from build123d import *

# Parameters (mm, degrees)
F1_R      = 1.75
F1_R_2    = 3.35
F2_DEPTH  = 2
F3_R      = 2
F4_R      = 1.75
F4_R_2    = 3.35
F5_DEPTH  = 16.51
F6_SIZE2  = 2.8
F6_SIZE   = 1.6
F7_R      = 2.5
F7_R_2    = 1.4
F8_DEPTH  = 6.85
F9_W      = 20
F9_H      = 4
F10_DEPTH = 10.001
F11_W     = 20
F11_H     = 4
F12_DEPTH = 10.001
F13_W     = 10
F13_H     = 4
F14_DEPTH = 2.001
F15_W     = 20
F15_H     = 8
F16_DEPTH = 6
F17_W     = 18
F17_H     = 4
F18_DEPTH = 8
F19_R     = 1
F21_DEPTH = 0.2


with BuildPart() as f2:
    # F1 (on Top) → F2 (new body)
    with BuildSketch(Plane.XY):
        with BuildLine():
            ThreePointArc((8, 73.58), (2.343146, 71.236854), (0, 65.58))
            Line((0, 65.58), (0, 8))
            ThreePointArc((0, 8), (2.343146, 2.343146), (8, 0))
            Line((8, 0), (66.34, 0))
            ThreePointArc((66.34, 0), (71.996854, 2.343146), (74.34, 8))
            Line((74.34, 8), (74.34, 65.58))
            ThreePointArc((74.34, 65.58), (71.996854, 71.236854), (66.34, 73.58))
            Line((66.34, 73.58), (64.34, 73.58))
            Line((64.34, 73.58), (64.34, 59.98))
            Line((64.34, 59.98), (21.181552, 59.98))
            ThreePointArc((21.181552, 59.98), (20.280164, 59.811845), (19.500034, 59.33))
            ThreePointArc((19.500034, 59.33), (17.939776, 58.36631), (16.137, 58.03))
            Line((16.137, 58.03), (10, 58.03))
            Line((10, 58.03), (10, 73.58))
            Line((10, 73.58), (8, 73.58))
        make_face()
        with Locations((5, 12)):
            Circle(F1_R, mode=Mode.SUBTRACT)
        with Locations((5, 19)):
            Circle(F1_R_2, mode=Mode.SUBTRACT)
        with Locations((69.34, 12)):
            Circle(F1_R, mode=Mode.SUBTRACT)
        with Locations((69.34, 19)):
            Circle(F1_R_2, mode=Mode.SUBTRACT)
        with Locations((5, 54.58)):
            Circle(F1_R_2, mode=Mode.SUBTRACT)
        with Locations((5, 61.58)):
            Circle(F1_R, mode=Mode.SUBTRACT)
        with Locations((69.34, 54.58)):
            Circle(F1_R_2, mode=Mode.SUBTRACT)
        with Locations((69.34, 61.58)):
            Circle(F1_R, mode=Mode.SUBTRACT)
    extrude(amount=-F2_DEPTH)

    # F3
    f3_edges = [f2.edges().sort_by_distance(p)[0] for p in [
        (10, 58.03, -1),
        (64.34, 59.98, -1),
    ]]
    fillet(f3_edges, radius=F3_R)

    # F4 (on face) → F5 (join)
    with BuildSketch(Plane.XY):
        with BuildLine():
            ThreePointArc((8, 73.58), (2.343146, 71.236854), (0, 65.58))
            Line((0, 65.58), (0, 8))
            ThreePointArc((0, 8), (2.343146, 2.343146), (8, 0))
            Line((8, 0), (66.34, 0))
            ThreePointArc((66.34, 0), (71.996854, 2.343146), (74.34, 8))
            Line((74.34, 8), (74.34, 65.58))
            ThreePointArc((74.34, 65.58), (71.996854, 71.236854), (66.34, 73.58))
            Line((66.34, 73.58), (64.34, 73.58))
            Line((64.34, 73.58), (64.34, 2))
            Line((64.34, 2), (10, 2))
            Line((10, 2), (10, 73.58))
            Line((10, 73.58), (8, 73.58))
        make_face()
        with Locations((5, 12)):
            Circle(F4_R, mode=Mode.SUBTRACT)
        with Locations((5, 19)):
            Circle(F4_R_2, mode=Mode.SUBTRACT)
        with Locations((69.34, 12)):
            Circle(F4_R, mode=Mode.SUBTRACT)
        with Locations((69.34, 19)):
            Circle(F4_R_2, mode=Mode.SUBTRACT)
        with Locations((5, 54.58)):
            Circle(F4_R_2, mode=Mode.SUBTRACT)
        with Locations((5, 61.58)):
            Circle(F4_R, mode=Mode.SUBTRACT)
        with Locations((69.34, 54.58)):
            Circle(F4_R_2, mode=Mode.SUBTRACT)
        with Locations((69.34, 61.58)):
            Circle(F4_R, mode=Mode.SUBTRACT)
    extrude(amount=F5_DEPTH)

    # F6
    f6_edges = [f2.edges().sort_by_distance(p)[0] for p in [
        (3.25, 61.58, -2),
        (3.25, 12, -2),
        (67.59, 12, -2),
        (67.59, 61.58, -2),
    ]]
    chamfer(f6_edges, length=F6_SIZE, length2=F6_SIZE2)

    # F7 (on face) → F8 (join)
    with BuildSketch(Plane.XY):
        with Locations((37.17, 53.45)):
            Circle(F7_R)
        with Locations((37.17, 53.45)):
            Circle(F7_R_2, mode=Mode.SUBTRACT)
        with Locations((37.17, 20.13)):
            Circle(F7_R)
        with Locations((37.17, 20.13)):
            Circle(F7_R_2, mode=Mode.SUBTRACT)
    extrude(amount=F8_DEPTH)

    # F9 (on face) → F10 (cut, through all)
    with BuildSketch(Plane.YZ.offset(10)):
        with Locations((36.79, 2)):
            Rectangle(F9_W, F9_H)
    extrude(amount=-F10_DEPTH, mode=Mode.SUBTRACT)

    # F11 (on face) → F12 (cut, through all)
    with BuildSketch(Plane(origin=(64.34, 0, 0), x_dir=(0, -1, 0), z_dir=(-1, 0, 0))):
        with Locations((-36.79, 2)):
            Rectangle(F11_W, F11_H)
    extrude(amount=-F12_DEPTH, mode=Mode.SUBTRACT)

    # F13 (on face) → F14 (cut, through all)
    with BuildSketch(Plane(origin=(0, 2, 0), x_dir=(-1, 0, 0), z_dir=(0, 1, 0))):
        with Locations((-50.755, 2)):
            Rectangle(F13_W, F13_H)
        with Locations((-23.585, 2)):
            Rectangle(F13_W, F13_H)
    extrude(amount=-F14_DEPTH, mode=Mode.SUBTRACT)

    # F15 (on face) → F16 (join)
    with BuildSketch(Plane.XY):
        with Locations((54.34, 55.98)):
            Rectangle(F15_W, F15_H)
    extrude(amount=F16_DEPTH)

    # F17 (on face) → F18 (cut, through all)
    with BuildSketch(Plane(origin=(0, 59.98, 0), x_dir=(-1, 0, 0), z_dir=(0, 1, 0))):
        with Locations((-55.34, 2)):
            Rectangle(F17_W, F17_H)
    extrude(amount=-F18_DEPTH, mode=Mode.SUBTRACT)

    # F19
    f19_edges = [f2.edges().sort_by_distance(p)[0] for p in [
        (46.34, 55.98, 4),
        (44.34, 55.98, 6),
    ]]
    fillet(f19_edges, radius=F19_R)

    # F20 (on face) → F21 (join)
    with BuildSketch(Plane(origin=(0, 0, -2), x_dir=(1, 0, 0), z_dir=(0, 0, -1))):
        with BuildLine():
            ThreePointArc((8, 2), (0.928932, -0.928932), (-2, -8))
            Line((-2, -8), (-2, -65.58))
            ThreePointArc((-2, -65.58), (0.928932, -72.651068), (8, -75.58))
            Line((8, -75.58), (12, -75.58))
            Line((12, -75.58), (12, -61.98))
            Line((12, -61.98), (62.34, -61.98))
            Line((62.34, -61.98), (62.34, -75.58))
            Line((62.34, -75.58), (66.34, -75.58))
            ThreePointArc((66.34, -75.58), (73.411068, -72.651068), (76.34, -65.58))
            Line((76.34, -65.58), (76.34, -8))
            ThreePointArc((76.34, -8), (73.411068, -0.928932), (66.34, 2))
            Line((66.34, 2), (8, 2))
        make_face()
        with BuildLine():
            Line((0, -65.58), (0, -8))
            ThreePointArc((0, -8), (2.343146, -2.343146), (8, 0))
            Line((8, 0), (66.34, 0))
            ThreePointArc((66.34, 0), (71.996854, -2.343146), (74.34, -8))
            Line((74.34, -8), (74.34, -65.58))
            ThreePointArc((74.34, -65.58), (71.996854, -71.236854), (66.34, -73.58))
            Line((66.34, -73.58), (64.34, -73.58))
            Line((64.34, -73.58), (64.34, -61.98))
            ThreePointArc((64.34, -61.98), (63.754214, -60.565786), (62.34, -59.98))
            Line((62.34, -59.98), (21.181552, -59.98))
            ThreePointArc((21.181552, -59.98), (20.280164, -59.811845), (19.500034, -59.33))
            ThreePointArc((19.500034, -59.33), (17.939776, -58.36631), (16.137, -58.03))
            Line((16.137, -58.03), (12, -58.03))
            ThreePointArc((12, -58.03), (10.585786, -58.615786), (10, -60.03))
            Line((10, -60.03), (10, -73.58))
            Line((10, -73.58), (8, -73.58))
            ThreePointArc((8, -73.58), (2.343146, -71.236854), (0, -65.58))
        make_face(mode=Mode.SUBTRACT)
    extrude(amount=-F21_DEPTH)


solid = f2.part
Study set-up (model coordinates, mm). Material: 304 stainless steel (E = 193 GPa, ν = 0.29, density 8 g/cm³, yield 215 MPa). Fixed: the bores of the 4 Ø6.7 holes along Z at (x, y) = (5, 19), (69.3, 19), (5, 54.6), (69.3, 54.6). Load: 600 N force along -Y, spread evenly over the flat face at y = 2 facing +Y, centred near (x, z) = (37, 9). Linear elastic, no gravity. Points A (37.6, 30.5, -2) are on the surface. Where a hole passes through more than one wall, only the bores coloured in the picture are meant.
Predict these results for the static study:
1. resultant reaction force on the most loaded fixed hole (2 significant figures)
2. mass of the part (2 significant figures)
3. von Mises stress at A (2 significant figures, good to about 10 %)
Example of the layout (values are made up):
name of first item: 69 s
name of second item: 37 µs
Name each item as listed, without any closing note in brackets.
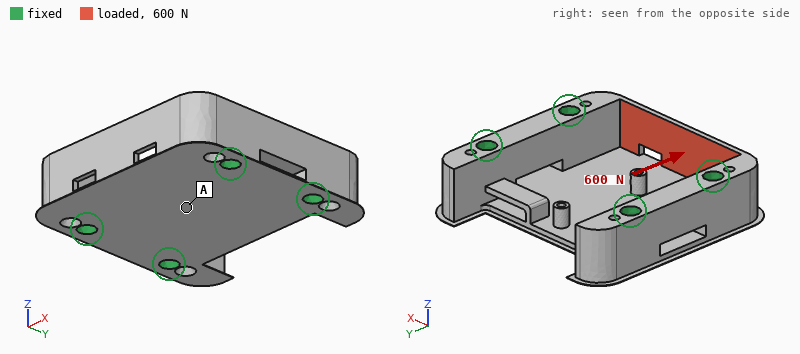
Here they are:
resultant reaction force on the most loaded fixed hole: 260 N
mass of the part: 240 g
von Mises stress at A: 8.0 MPa
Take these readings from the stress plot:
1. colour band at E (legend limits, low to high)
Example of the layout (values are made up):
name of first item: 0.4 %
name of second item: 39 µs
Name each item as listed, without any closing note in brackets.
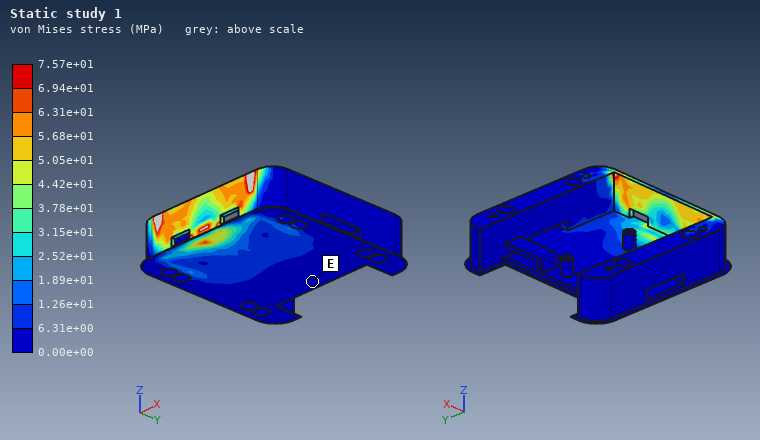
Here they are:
colour band at E: 0.00e+00 to 6.31e+00 MPa
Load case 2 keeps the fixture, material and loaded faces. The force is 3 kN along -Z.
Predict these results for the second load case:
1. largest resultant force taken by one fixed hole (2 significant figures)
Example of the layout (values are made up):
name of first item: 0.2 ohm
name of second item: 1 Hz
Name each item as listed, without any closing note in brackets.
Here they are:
largest resultant force taken by one fixed hole: 1.5 kN
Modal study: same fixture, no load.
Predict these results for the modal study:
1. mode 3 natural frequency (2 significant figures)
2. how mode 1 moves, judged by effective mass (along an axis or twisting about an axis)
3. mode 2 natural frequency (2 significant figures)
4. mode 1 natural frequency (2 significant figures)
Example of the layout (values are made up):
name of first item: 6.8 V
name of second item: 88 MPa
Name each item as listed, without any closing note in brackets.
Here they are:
mode 3 natural frequency: 6000 Hz
how mode 1 moves, judged by effective mass: along Z
mode 2 natural frequency: 4900 Hz
mode 1 natural frequency: 3500 Hz
